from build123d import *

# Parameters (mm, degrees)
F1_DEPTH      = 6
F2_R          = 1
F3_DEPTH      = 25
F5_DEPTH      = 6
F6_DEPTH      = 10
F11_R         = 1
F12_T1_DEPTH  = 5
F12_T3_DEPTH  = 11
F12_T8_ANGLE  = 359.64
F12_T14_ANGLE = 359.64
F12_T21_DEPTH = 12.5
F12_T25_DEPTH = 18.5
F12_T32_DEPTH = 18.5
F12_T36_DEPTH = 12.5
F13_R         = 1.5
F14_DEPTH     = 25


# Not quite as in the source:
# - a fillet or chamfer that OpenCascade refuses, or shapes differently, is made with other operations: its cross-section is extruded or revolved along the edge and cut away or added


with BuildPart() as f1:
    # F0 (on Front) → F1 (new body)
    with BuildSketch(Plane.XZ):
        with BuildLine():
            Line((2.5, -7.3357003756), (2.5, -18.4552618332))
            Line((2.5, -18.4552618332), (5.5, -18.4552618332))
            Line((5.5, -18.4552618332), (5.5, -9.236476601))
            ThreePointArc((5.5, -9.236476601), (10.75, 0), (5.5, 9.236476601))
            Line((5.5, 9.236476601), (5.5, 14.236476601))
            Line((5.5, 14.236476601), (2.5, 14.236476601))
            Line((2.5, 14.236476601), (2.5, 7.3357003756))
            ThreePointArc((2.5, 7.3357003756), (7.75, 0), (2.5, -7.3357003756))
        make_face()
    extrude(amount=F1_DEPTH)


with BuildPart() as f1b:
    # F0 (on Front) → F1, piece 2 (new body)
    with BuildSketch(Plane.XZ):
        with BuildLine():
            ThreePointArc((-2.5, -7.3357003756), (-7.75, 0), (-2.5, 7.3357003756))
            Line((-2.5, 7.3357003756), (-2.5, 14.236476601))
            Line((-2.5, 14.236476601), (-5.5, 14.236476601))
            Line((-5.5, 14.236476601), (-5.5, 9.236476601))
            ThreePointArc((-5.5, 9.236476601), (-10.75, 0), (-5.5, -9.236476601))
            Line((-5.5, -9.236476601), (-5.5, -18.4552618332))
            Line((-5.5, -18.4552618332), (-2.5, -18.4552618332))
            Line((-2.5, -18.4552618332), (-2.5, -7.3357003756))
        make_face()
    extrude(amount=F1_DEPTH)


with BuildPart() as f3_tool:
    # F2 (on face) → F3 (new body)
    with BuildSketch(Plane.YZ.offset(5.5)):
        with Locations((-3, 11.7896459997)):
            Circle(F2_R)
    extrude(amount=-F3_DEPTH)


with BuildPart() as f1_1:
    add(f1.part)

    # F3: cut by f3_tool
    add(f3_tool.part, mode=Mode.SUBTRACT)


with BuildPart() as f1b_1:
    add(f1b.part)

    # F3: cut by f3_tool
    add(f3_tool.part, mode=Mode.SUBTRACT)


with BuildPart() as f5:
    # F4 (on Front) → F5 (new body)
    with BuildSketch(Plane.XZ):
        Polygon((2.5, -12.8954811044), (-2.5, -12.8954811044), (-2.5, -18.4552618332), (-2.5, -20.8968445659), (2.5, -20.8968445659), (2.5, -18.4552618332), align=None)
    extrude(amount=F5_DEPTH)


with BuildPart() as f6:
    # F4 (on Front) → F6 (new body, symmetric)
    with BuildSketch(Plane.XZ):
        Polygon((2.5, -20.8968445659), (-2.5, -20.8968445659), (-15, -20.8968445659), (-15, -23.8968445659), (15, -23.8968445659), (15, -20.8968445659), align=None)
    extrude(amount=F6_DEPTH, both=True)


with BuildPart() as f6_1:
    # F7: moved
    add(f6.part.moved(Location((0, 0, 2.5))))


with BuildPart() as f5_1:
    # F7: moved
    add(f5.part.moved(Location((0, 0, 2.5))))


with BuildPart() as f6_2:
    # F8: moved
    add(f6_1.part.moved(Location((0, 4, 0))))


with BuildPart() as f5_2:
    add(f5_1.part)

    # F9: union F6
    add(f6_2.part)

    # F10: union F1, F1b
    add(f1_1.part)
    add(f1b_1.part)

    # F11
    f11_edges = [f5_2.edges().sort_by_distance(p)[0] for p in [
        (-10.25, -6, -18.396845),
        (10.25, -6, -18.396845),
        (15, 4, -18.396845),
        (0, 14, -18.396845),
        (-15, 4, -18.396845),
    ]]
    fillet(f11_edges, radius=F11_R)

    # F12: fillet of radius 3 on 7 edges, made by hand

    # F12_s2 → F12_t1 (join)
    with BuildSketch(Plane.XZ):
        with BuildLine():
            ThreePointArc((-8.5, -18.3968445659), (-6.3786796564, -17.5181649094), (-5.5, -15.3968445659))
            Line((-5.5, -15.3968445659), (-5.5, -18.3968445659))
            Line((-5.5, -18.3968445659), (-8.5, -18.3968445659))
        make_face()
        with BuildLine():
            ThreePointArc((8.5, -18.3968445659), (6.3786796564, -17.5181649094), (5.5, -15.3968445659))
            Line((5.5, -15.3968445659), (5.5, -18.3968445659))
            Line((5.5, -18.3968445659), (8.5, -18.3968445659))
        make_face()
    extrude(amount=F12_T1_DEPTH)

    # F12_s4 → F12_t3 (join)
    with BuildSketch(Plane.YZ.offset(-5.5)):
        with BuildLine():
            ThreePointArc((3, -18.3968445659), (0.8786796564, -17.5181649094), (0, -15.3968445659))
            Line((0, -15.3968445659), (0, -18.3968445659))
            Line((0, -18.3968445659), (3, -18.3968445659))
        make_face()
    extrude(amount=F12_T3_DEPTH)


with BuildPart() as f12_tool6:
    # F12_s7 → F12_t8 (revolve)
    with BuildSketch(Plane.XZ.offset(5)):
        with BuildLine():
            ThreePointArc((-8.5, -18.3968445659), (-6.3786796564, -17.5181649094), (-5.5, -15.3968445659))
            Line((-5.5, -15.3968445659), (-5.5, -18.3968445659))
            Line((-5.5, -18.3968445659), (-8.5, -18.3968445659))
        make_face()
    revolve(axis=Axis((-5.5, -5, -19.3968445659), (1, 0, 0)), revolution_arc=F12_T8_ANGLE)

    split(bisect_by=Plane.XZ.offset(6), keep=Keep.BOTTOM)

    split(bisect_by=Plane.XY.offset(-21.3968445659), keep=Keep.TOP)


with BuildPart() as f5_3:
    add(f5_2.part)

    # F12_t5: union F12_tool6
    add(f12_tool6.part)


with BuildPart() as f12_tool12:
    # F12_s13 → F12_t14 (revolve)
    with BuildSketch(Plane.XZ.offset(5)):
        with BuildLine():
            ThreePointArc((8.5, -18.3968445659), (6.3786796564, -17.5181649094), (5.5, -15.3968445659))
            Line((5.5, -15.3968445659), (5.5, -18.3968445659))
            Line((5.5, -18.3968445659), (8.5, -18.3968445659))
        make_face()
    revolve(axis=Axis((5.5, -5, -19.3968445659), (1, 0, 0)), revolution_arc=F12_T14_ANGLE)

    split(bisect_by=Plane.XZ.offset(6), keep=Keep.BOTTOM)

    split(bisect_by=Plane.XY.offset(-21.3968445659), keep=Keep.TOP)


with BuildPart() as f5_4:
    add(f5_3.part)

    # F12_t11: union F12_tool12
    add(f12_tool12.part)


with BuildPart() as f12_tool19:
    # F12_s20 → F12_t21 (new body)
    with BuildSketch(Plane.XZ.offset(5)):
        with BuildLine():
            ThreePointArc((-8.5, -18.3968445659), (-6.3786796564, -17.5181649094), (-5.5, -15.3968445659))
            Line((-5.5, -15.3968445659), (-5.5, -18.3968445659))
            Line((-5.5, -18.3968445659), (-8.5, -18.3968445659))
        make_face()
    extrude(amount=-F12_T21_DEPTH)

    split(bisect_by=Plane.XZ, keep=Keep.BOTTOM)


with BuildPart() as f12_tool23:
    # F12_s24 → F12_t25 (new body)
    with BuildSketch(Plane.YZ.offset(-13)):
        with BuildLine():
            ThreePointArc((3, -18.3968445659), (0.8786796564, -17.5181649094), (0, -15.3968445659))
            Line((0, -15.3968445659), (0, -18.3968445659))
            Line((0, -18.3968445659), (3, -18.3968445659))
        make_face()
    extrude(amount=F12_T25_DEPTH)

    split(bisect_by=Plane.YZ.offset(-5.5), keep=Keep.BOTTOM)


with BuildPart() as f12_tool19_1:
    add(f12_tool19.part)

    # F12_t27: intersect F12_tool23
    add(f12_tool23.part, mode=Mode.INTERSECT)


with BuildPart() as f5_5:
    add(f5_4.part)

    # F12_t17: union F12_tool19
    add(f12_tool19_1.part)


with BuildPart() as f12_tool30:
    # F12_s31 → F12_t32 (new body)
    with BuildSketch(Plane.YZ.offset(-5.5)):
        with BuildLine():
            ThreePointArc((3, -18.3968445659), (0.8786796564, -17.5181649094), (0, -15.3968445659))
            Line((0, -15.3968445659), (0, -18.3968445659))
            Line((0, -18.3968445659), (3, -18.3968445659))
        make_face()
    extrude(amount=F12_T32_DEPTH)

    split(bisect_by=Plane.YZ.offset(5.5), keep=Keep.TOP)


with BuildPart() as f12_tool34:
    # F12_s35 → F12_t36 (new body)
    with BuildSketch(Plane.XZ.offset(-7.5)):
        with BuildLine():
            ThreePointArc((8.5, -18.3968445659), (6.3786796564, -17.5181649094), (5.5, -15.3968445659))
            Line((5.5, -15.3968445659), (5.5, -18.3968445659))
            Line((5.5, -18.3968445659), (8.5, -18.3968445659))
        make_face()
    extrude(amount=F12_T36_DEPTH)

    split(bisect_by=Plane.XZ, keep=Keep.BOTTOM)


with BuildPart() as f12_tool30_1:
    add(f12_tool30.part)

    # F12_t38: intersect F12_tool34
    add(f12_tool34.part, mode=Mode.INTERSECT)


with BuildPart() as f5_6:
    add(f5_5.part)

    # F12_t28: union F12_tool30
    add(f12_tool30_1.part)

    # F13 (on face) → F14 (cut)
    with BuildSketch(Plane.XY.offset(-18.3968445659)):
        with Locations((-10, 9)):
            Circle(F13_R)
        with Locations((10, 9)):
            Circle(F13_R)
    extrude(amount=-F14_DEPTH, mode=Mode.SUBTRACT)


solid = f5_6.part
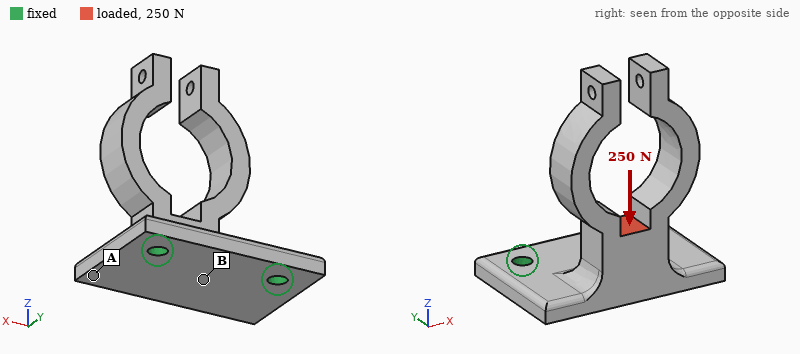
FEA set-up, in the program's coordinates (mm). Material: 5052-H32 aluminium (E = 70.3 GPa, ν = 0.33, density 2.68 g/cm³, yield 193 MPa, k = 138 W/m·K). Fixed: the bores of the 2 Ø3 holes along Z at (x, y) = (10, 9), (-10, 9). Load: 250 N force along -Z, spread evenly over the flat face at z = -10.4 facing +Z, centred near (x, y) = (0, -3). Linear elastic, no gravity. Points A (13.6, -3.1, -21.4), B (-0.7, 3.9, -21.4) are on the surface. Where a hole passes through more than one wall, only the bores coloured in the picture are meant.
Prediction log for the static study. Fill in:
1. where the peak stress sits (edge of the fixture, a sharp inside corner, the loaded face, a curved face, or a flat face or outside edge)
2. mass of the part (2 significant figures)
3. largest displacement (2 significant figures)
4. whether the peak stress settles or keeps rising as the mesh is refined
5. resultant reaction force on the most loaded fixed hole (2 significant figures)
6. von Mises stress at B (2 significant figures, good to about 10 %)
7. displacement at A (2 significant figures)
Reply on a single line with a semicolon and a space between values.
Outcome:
edge of the fixture; 8.9 g; 0.14 mm; keeps rising; 130 N; 29 MPa; 0.030 mm
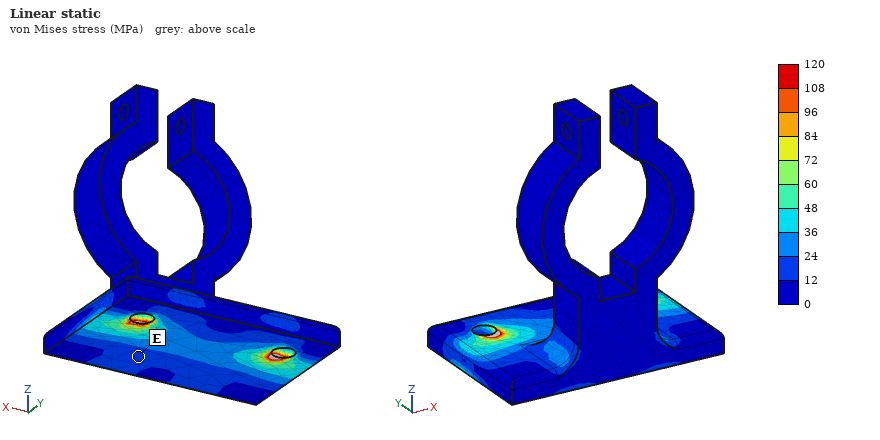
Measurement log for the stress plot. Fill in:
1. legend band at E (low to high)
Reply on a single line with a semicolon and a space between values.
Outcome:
12 to 24 MPa
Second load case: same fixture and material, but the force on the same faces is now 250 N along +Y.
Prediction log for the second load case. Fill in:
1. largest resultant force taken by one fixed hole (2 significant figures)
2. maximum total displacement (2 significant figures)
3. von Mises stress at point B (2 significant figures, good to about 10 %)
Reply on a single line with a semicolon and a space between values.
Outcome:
140 N; 0.19 mm; 44 MPa
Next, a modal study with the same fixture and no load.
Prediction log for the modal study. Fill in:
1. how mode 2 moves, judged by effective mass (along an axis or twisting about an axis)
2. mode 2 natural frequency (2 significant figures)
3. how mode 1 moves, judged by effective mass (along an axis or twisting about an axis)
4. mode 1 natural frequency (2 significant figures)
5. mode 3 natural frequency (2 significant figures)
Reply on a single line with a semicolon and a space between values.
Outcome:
along X; 2800 Hz; along Y; 2300 Hz; 3200 Hz
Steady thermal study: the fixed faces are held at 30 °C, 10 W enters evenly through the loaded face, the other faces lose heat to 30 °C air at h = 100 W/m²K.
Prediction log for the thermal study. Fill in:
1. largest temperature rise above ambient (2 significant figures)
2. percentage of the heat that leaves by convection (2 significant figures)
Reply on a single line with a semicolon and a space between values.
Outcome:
19 K; 22 %
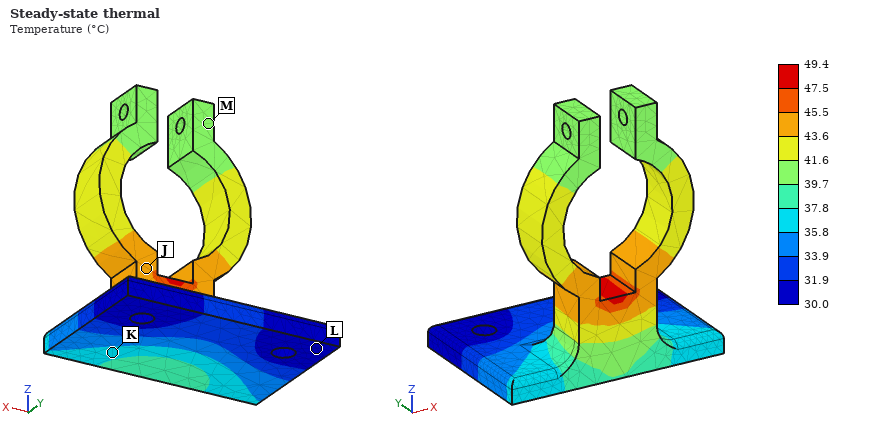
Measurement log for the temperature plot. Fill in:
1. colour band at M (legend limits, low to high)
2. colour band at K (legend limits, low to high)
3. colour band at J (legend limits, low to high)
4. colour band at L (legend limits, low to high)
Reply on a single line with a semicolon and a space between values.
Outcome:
39.7 to 41.6 °C; 35.8 to 37.8 °C; 43.6 to 45.5 °C; 30.0 to 31.9 °C
